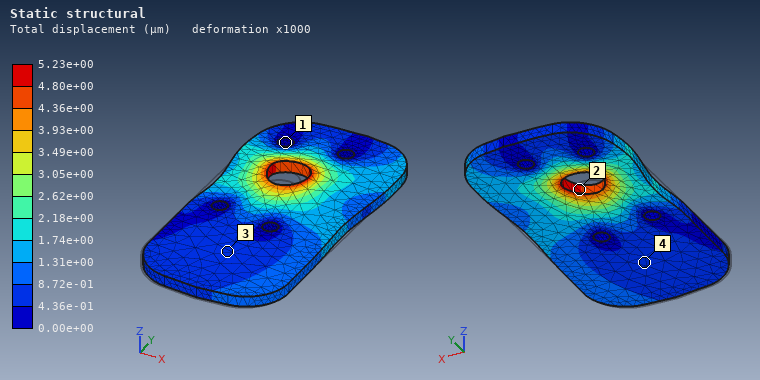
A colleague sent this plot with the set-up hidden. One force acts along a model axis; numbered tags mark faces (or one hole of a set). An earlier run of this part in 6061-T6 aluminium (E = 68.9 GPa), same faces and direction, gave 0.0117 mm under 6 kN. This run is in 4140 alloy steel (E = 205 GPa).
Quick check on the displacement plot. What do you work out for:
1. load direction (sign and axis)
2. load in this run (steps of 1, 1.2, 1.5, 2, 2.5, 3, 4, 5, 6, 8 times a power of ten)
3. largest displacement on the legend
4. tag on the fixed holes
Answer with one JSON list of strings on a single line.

["+Y", "8 kN", "5.23e+00 µm", "1"]
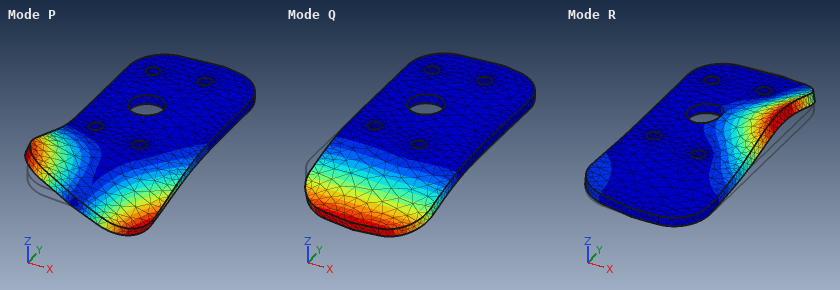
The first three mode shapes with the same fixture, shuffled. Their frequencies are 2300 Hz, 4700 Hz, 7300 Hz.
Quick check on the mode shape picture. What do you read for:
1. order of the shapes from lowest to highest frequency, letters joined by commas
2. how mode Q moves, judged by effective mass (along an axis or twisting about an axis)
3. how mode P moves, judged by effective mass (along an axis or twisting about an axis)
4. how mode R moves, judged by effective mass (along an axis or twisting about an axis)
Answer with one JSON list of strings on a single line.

["Q, P, R", "along Z", "twisting about Y", "along Z"]
